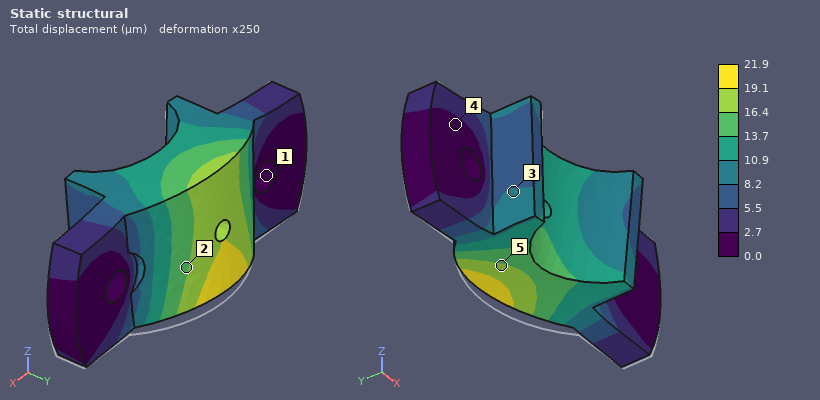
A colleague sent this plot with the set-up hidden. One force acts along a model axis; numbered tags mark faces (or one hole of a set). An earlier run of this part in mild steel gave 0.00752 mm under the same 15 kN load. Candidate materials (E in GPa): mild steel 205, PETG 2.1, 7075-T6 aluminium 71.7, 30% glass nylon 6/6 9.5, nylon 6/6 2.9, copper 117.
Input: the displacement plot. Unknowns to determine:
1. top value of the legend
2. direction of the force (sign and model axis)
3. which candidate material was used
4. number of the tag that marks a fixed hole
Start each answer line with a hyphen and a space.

- 21.9 µm
- +Z
- 7075-T6 aluminium
- 1
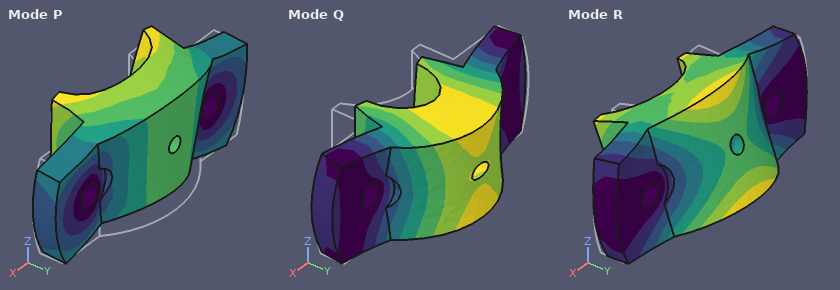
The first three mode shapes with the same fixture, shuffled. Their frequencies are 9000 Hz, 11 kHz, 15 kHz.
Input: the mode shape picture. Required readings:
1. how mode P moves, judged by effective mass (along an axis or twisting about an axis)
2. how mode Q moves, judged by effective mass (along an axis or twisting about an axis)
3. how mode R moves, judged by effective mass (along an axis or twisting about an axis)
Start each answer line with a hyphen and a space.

- along Z
- along Y
- twisting about X
